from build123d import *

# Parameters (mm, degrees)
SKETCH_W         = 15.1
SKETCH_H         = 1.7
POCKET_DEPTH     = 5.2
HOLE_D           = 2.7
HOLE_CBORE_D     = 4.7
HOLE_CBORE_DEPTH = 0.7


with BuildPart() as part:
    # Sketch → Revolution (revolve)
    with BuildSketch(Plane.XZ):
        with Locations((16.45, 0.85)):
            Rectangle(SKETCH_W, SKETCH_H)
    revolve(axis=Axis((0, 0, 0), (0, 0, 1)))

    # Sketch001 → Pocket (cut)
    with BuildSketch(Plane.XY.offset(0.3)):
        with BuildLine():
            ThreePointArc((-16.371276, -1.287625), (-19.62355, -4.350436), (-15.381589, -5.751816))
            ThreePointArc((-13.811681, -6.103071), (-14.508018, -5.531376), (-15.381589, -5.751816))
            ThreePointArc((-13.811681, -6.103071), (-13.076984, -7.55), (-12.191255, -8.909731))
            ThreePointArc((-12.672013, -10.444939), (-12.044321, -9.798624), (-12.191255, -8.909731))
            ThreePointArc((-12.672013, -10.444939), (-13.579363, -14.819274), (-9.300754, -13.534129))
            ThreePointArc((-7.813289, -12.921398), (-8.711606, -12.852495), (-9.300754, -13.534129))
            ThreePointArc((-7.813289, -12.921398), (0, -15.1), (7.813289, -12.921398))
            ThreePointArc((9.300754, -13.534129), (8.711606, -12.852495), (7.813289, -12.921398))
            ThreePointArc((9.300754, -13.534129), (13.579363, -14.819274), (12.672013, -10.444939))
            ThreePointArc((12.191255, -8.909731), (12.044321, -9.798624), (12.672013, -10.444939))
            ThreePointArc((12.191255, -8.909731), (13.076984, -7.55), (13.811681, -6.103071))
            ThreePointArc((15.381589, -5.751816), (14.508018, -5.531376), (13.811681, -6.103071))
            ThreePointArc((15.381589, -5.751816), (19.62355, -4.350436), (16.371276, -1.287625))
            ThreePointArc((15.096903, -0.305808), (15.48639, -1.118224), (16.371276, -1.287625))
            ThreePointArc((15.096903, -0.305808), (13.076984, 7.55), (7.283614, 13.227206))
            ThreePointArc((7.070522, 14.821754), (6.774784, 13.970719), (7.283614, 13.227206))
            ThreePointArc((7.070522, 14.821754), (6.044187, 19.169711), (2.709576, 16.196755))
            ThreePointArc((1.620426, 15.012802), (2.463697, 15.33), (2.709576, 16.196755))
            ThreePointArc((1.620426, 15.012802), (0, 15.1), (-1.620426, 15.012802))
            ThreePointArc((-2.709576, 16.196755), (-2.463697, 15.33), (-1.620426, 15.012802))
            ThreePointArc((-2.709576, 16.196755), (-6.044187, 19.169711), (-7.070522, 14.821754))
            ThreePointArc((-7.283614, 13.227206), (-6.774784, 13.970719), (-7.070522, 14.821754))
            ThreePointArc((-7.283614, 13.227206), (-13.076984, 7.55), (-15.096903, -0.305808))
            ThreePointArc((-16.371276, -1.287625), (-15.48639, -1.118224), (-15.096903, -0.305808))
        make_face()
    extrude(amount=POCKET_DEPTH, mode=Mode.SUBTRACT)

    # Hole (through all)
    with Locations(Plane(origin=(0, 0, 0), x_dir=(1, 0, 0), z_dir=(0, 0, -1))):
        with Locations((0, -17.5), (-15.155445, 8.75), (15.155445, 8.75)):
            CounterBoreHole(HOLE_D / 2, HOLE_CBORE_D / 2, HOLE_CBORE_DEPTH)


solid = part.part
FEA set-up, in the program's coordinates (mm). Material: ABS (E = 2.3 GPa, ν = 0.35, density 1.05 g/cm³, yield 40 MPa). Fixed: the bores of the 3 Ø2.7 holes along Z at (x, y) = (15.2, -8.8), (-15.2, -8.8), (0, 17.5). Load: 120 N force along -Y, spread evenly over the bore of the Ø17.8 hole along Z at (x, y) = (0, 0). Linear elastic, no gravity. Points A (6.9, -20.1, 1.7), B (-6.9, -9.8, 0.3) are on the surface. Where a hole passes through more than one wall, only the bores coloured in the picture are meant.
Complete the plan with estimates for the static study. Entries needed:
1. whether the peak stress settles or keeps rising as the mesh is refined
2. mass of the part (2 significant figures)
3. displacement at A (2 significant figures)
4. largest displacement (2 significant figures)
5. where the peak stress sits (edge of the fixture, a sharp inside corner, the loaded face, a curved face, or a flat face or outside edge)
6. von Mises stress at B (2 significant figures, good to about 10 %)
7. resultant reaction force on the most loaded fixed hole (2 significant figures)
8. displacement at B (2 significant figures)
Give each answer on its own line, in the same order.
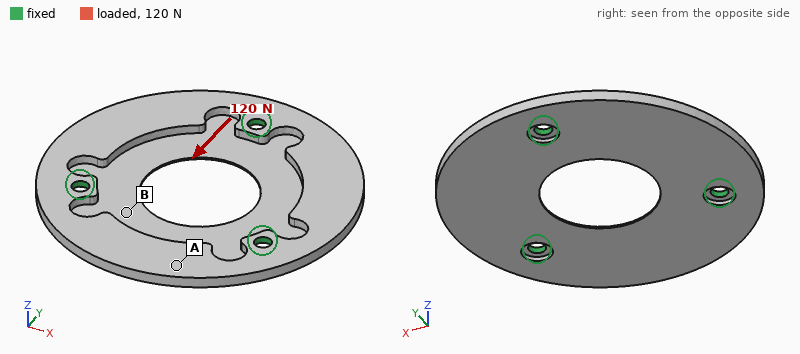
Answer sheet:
keeps rising
1.8 g
0.15 mm
0.25 mm
a sharp inside corner
6.3 MPa
41 N
0.10 mm
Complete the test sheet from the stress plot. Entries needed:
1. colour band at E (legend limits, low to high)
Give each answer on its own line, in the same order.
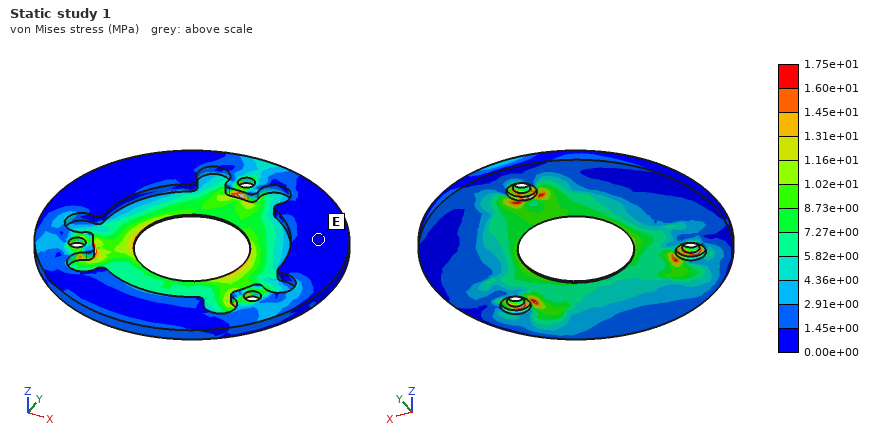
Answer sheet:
0.00e+00 to 1.45e+00 MPa
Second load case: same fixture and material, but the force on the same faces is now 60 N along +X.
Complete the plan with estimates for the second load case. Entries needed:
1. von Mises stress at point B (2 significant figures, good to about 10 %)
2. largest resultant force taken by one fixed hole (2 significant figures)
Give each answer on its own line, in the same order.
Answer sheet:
4.3 MPa
21 N
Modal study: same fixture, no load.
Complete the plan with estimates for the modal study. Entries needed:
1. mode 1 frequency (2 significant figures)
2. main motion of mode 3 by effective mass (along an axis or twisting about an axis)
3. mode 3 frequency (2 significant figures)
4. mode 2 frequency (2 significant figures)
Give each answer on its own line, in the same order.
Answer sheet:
970 Hz
along Z
1100 Hz
970 Hz
